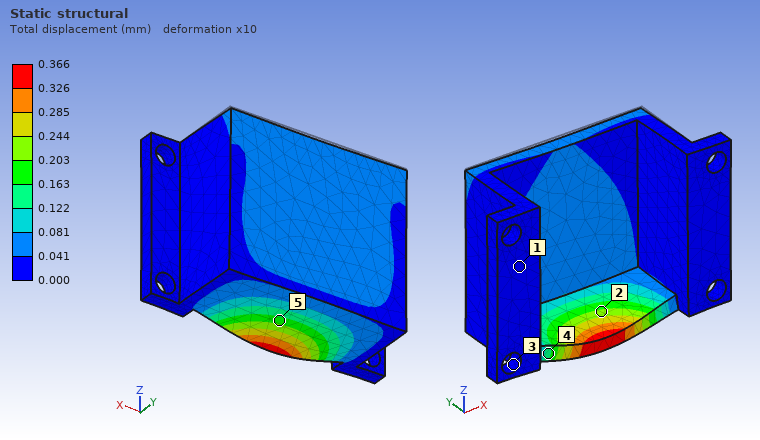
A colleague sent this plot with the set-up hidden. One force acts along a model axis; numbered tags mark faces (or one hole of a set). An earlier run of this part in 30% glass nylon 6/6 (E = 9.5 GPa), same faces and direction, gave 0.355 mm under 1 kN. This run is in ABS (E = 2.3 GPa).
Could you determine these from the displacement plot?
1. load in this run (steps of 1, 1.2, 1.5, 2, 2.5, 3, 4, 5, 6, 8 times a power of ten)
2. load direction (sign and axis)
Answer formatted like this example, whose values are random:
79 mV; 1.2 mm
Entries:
250 N; -Z
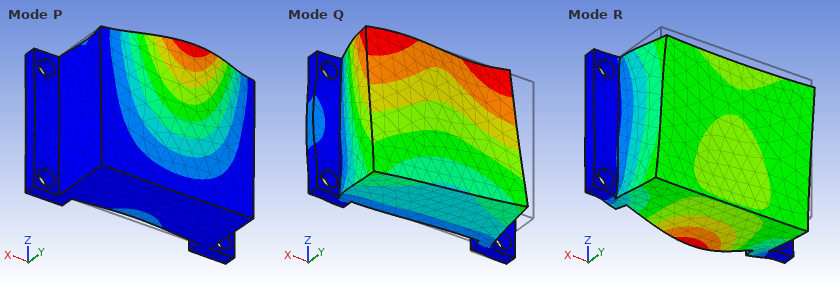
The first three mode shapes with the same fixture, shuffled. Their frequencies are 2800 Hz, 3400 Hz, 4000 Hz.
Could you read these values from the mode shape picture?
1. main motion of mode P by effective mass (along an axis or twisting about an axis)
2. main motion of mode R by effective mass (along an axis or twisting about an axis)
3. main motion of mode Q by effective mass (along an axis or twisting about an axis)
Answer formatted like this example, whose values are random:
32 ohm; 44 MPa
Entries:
along Y; along Z; along X
